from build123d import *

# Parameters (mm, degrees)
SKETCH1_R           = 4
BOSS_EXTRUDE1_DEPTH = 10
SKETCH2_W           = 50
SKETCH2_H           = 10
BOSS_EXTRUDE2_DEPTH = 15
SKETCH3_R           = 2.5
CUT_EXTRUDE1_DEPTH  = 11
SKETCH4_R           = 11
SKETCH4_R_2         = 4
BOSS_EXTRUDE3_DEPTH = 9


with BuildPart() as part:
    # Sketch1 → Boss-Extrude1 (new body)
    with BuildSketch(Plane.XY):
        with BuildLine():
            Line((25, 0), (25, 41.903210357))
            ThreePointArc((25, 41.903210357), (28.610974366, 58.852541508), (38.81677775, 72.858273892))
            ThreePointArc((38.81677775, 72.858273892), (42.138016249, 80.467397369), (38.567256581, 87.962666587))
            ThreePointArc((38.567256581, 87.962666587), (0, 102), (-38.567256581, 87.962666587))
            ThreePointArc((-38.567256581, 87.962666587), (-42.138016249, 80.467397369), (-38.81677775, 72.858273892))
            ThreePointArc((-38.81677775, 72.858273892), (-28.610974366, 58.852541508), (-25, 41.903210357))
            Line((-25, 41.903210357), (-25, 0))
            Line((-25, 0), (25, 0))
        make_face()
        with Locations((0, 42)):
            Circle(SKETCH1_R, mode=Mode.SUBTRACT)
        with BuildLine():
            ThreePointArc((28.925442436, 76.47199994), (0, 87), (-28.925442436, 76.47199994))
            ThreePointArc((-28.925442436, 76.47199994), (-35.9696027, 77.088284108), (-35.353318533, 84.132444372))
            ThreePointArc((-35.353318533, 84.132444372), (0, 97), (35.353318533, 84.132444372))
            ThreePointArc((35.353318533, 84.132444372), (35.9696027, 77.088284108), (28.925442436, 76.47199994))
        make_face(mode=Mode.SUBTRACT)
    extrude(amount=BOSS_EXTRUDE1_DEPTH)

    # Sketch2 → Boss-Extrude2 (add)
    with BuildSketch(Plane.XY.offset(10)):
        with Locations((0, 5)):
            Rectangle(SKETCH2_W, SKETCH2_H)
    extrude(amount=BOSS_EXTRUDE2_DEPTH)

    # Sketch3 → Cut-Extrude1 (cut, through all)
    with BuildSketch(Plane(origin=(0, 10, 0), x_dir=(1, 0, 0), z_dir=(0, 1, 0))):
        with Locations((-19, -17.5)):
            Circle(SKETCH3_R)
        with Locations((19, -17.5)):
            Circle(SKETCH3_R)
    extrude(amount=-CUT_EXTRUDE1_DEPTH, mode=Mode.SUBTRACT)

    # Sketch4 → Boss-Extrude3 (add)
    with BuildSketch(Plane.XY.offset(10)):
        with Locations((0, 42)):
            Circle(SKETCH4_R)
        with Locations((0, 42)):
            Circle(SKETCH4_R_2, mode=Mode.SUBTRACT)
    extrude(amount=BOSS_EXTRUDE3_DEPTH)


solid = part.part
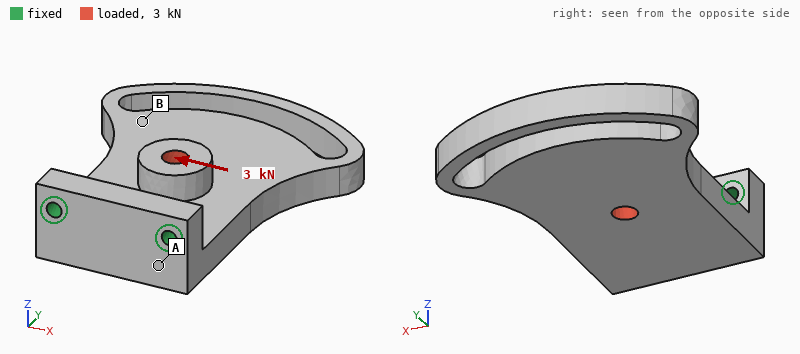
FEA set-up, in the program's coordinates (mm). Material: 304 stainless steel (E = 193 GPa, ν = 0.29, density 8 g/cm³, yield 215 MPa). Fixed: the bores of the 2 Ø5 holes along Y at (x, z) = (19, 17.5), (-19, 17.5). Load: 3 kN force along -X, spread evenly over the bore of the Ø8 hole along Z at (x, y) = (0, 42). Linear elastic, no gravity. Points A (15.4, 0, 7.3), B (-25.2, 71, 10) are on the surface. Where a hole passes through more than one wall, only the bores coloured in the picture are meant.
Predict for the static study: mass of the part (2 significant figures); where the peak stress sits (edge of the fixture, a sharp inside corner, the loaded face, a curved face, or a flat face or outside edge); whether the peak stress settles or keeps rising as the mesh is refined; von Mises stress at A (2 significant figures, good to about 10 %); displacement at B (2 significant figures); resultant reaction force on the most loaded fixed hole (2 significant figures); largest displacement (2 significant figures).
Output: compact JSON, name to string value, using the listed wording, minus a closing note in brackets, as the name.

{"mass of the part": "490 g", "where the peak stress sits": "edge of the fixture", "whether the peak stress settles or keeps rising as the mesh is refined": "keeps rising", "von Mises stress at A": "24 MPa", "displacement at B": "35 µm", "resultant reaction force on the most loaded fixed hole": "3.2 kN", "largest displacement": "45 µm"}
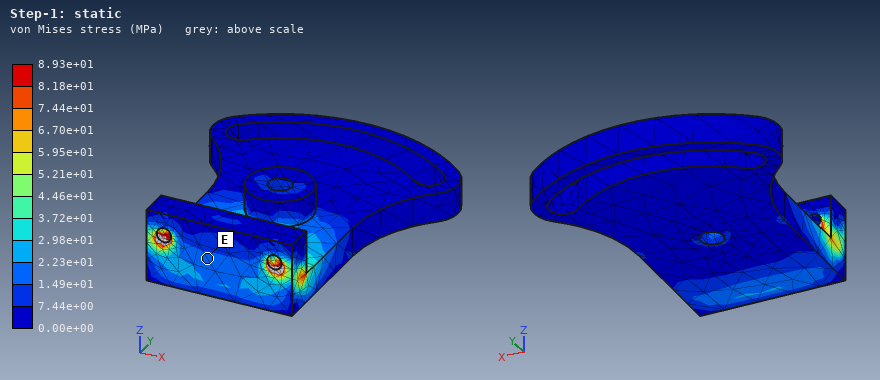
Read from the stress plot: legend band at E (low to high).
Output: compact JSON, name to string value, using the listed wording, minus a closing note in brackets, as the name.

{"legend band at E": "1.49e+01 to 2.23e+01 MPa"}
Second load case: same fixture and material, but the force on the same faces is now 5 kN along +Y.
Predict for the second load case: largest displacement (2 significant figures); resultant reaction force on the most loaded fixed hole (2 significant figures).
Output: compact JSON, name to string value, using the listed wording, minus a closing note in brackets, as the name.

{"largest displacement": "37 µm", "resultant reaction force on the most loaded fixed hole": "2.5 kN"}
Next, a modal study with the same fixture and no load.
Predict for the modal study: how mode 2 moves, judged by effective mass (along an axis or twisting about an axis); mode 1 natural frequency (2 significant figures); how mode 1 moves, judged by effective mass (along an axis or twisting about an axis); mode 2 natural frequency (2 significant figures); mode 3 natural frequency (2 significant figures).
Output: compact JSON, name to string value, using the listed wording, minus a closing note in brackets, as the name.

{"how mode 2 moves, judged by effective mass": "along X", "mode 1 natural frequency": "730 Hz", "how mode 1 moves, judged by effective mass": "along Z", "mode 2 natural frequency": "2100 Hz", "mode 3 natural frequency": "2600 Hz"}
